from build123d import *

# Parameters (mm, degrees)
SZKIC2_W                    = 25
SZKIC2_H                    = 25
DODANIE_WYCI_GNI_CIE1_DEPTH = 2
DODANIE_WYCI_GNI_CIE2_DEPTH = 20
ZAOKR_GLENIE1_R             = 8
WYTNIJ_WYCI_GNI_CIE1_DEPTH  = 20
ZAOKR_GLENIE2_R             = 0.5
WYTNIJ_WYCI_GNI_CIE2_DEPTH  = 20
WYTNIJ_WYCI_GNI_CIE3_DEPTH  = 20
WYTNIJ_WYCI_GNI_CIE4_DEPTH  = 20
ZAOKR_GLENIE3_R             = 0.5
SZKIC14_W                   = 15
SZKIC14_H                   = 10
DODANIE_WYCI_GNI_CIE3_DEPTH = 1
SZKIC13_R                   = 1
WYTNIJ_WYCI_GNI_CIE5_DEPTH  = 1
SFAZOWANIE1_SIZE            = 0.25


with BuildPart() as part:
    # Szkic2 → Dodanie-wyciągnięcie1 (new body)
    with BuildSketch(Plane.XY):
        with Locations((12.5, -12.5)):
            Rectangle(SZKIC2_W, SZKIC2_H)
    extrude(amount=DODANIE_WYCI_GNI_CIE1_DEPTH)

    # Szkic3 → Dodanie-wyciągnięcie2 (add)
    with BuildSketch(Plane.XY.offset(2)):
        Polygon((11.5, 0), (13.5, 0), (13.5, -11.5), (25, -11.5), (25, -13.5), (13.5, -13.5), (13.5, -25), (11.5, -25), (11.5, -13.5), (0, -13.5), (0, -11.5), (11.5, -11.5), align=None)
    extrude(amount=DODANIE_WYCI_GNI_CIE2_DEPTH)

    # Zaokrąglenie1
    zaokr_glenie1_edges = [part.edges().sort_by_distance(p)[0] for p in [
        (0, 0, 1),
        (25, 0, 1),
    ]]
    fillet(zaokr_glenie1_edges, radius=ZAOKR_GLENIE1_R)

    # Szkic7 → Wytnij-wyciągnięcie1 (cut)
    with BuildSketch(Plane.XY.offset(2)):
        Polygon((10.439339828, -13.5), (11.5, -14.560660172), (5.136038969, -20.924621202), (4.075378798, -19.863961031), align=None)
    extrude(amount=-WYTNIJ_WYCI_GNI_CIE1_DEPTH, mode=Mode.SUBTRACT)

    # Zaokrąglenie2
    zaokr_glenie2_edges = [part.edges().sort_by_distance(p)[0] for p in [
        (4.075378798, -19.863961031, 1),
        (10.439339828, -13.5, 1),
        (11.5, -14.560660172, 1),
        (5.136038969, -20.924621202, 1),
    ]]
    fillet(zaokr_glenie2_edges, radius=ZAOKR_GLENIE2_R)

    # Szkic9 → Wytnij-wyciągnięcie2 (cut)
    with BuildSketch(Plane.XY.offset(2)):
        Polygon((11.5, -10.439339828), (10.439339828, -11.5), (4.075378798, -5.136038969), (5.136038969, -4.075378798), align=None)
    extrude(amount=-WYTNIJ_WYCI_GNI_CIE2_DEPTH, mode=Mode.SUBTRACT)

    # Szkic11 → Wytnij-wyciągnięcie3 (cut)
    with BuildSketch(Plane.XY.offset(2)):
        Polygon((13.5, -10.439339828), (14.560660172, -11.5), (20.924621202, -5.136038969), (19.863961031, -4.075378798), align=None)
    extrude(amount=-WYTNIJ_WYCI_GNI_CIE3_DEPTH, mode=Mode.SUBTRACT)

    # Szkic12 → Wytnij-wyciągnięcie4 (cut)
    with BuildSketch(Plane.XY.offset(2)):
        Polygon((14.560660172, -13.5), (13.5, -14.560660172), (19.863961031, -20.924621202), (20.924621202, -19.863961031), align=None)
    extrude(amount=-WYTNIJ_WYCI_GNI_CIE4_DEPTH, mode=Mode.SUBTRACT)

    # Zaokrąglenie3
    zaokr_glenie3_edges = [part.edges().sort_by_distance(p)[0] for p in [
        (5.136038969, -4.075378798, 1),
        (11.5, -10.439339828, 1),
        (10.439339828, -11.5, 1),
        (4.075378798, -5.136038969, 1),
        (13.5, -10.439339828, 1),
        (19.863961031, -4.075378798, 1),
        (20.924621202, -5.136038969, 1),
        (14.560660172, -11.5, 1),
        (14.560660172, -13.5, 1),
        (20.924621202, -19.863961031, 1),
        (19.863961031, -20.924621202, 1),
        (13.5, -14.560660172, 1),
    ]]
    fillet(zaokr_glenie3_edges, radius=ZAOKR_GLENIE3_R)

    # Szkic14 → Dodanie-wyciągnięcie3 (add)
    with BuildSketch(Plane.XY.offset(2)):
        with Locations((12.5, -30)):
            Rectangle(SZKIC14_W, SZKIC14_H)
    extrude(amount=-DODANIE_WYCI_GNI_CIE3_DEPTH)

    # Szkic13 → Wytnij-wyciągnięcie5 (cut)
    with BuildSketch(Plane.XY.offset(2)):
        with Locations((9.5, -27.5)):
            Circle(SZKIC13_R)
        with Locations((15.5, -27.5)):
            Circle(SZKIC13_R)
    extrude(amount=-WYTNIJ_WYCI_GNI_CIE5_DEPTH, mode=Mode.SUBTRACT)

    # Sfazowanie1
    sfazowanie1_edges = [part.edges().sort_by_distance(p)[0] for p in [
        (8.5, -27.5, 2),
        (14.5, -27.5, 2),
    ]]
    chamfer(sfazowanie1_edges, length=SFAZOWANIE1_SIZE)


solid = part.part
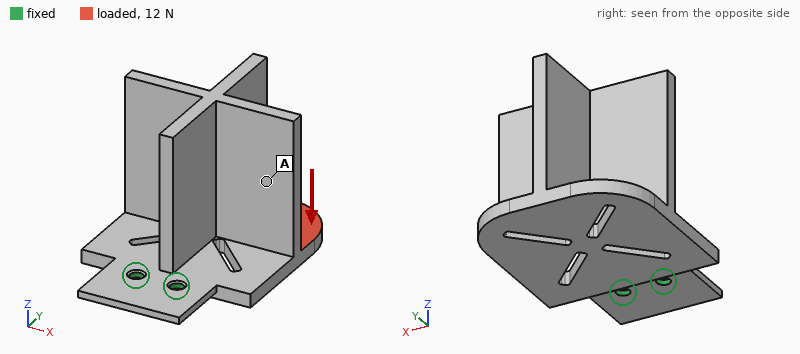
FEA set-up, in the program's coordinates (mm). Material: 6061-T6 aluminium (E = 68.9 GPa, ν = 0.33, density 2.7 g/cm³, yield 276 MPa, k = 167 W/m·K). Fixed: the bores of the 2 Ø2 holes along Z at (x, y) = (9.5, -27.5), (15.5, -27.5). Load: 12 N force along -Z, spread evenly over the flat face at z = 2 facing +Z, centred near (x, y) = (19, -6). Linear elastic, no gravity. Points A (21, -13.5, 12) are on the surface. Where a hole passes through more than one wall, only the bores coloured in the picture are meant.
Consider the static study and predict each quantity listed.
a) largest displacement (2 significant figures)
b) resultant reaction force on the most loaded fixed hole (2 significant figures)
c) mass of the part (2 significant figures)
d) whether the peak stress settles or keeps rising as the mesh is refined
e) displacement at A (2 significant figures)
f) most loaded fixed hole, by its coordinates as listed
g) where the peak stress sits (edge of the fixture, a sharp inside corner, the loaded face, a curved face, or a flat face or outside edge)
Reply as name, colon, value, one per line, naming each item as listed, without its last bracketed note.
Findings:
largest displacement: 0.25 mm
resultant reaction force on the most loaded fixed hole: 16 N
mass of the part: 8.5 g
whether the peak stress settles or keeps rising as the mesh is refined: keeps rising
displacement at A: 0.13 mm
most loaded fixed hole, by its coordinates as listed: (15.5, -27.5)
where the peak stress sits: edge of the fixture
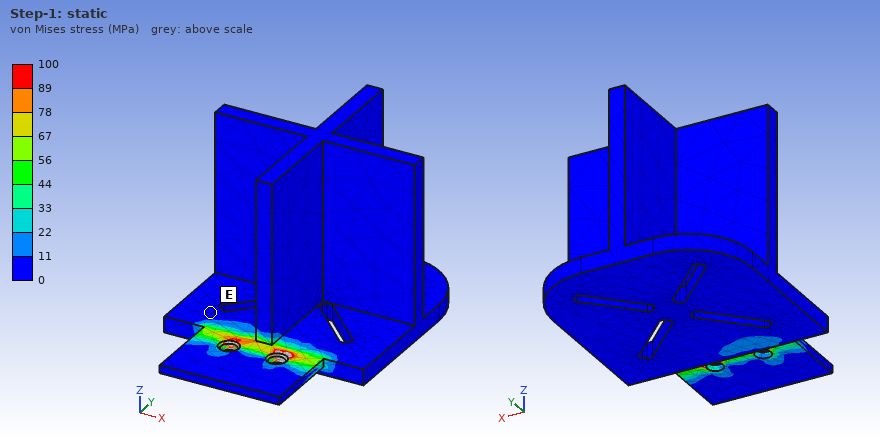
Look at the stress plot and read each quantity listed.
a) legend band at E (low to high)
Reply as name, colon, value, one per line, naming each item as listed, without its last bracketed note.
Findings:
legend band at E: 0 to 11 MPa
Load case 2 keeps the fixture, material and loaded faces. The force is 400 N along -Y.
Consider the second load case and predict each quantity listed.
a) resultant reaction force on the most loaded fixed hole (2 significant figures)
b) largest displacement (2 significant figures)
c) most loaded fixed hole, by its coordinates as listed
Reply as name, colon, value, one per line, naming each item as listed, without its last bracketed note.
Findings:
resultant reaction force on the most loaded fixed hole: 560 N
largest displacement: 0.24 mm
most loaded fixed hole, by its coordinates as listed: (15.5, -27.5)
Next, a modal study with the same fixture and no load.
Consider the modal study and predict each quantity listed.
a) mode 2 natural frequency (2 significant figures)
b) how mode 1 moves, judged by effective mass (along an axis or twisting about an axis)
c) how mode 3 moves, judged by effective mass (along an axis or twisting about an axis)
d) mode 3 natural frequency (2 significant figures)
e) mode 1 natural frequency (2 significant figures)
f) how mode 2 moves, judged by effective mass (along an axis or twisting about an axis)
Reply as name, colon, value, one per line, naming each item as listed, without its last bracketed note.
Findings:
mode 2 natural frequency: 1500 Hz
how mode 1 moves, judged by effective mass: along Z
how mode 3 moves, judged by effective mass: along X
mode 3 natural frequency: 5200 Hz
mode 1 natural frequency: 570 Hz
how mode 2 moves, judged by effective mass: along X
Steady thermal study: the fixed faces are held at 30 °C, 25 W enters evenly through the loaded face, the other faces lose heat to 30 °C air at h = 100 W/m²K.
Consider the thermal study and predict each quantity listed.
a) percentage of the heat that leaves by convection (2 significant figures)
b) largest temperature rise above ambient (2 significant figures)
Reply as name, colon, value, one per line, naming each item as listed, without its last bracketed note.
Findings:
percentage of the heat that leaves by convection: 48 %
largest temperature rise above ambient: 71 K
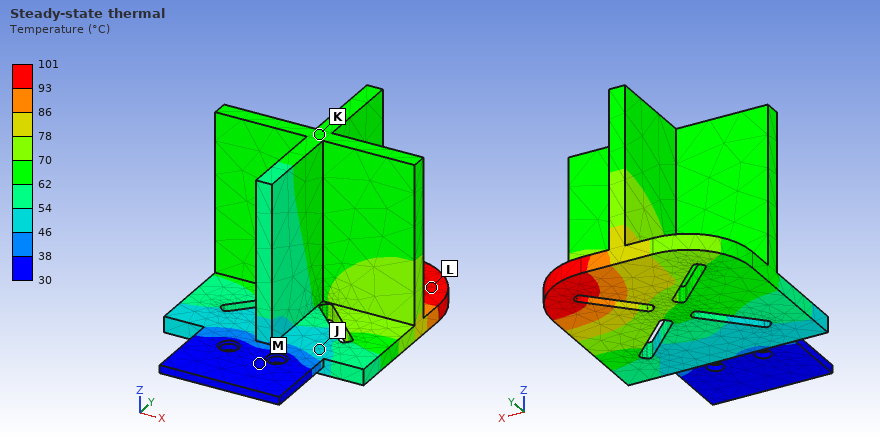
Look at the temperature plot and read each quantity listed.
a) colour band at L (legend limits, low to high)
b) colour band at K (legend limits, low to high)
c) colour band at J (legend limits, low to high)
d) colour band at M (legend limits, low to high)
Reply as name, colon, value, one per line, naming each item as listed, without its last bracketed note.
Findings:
colour band at L: 93 to 101 °C
colour band at K: 62 to 70 °C
colour band at J: 46 to 54 °C
colour band at M: 30 to 38 °C
